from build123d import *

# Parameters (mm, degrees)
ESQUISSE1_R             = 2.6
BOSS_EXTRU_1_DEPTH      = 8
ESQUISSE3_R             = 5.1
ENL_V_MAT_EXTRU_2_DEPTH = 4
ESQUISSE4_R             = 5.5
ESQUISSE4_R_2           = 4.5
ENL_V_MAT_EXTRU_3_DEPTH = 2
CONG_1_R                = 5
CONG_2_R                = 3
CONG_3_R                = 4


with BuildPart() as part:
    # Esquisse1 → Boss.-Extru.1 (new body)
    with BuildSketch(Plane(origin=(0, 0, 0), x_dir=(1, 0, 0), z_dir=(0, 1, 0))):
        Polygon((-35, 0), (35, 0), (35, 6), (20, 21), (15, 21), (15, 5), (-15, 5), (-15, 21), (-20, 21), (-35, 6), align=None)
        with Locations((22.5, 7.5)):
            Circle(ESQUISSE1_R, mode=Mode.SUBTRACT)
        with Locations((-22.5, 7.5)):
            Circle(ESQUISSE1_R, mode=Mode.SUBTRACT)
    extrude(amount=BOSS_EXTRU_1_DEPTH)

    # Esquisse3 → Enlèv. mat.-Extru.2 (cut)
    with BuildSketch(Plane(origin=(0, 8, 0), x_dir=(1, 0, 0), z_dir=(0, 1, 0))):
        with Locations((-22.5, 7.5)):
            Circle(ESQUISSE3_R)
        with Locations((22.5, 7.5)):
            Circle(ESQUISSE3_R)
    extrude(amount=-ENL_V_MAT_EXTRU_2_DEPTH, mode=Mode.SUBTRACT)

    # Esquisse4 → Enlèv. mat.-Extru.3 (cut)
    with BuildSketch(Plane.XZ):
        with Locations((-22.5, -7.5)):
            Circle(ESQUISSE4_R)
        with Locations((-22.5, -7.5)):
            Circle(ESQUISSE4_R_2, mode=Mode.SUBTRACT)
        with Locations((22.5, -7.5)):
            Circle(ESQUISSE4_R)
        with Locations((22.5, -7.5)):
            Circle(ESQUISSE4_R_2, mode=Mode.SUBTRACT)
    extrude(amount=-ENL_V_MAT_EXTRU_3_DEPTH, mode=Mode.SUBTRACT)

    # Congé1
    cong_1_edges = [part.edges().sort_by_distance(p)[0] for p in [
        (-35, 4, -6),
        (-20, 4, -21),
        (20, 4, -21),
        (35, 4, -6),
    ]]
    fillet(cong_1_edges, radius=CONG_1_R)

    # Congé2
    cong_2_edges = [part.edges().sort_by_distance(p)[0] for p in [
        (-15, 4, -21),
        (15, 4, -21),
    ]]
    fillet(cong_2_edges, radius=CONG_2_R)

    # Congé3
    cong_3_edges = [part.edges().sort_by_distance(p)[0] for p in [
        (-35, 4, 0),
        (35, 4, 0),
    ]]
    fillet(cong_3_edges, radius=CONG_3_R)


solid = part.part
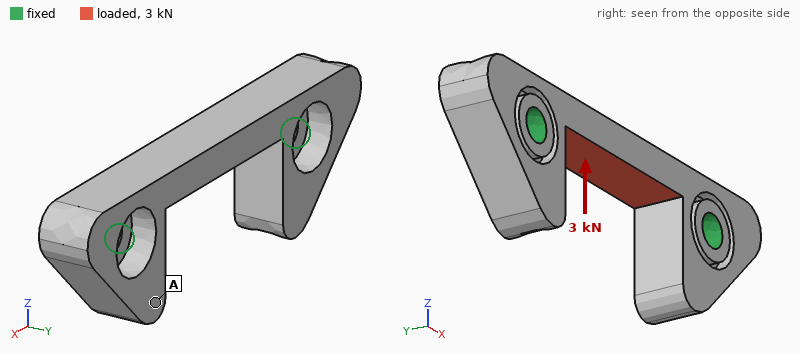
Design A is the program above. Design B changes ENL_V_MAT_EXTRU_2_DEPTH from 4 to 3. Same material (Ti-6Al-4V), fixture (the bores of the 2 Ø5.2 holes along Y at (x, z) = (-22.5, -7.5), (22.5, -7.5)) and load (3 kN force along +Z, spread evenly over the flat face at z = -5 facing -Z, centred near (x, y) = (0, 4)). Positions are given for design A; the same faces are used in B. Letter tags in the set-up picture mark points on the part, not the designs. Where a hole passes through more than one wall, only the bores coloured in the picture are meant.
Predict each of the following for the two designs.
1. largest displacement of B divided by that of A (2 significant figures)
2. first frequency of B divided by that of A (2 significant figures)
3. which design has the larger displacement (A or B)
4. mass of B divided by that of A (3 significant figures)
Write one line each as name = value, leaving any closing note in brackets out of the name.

largest displacement of B divided by that of A = 0.90
first frequency of B divided by that of A = 1.1
which design has the larger displacement = A
mass of B divided by that of A = 1.02
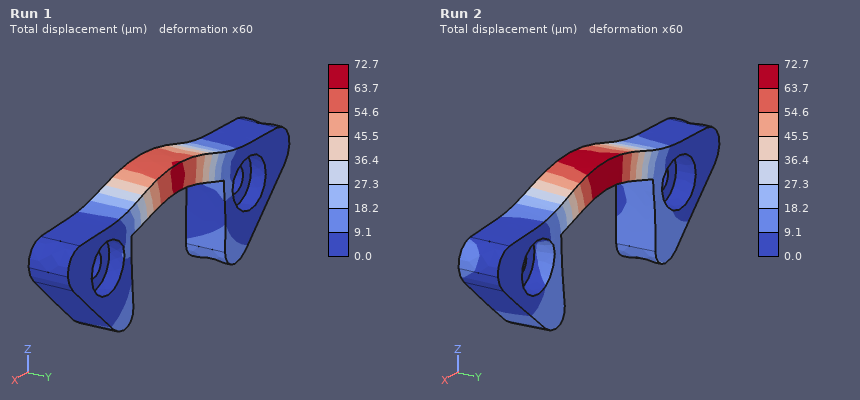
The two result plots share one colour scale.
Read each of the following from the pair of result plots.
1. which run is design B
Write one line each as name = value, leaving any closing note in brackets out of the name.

which run is design B = Run 1
